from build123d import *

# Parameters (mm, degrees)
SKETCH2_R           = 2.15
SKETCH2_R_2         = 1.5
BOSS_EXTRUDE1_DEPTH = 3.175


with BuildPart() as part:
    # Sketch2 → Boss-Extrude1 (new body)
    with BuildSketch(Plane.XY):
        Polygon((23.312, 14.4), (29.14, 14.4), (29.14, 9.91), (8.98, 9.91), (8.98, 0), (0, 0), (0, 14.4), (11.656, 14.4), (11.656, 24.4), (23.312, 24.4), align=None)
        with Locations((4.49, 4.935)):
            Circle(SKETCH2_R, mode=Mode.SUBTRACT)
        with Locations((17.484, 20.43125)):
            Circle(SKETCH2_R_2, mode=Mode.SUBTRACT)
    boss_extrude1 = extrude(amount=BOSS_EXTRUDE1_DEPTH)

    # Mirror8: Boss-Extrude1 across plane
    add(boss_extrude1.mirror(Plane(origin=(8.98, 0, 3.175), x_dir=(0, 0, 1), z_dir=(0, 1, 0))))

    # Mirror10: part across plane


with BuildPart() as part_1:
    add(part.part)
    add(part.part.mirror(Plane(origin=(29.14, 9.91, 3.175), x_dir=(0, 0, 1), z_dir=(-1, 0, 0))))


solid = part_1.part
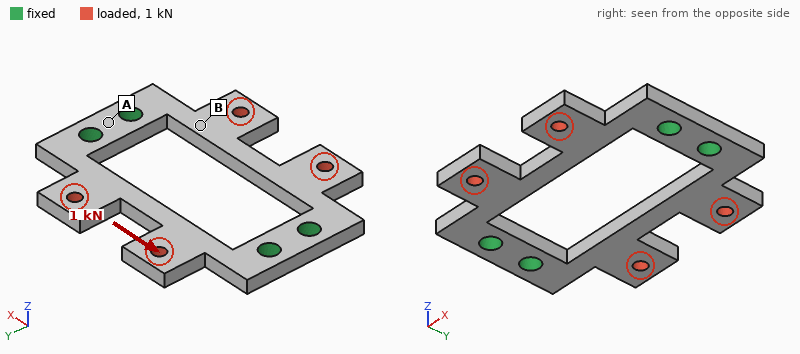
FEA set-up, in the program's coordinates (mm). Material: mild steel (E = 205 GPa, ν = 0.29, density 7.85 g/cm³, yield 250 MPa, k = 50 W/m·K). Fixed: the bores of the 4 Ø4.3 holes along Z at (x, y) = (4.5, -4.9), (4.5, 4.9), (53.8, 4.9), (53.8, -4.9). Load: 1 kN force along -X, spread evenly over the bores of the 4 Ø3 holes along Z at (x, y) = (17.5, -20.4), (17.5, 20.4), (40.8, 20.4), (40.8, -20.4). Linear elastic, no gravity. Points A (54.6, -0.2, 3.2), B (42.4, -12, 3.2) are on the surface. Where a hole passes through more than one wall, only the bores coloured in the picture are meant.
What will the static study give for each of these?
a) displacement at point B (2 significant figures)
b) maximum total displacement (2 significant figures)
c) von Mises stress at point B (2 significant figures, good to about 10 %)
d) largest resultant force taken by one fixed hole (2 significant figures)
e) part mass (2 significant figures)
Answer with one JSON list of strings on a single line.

["2.2 µm", "6.6 µm", "13 MPa", "270 N", "31 g"]
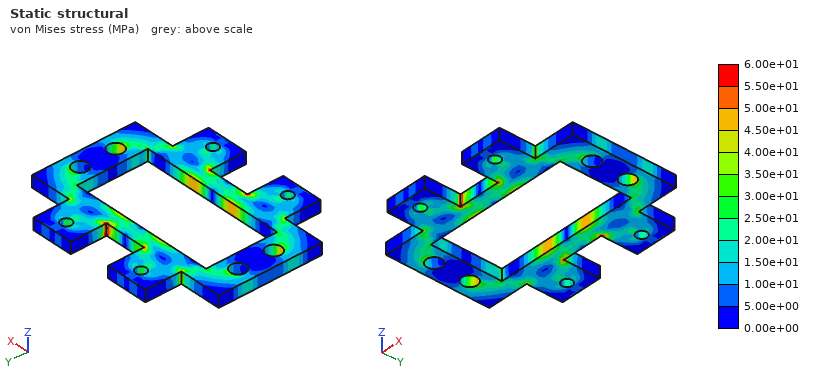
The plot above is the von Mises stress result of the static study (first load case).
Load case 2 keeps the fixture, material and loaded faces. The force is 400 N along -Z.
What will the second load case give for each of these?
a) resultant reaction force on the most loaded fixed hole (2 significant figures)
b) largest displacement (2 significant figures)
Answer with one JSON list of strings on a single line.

["100 N", "86 µm"]
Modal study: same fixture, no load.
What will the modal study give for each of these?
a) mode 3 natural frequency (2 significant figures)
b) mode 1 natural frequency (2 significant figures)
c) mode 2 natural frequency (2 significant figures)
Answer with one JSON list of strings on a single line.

["6800 Hz", "3800 Hz", "3800 Hz"]
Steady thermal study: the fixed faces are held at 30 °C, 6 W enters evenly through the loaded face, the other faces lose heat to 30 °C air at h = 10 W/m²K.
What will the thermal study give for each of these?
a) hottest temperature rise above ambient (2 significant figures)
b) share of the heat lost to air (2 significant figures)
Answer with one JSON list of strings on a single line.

["27 K", "9.1 %"]
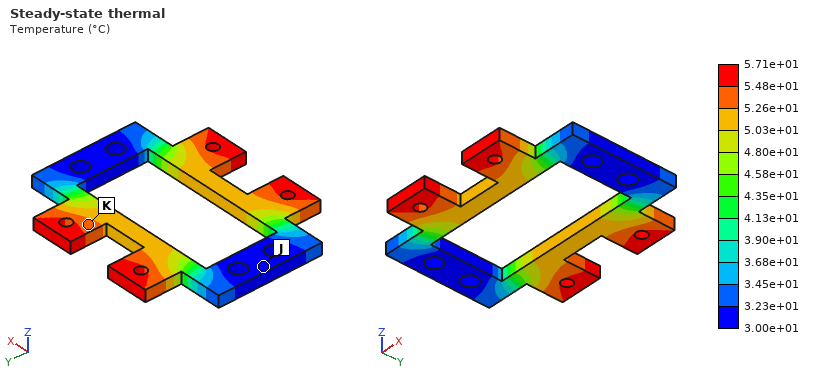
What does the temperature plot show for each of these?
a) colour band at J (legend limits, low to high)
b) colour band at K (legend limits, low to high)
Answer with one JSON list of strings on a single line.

["3.00e+01 to 3.23e+01 °C", "5.26e+01 to 5.48e+01 °C"]
